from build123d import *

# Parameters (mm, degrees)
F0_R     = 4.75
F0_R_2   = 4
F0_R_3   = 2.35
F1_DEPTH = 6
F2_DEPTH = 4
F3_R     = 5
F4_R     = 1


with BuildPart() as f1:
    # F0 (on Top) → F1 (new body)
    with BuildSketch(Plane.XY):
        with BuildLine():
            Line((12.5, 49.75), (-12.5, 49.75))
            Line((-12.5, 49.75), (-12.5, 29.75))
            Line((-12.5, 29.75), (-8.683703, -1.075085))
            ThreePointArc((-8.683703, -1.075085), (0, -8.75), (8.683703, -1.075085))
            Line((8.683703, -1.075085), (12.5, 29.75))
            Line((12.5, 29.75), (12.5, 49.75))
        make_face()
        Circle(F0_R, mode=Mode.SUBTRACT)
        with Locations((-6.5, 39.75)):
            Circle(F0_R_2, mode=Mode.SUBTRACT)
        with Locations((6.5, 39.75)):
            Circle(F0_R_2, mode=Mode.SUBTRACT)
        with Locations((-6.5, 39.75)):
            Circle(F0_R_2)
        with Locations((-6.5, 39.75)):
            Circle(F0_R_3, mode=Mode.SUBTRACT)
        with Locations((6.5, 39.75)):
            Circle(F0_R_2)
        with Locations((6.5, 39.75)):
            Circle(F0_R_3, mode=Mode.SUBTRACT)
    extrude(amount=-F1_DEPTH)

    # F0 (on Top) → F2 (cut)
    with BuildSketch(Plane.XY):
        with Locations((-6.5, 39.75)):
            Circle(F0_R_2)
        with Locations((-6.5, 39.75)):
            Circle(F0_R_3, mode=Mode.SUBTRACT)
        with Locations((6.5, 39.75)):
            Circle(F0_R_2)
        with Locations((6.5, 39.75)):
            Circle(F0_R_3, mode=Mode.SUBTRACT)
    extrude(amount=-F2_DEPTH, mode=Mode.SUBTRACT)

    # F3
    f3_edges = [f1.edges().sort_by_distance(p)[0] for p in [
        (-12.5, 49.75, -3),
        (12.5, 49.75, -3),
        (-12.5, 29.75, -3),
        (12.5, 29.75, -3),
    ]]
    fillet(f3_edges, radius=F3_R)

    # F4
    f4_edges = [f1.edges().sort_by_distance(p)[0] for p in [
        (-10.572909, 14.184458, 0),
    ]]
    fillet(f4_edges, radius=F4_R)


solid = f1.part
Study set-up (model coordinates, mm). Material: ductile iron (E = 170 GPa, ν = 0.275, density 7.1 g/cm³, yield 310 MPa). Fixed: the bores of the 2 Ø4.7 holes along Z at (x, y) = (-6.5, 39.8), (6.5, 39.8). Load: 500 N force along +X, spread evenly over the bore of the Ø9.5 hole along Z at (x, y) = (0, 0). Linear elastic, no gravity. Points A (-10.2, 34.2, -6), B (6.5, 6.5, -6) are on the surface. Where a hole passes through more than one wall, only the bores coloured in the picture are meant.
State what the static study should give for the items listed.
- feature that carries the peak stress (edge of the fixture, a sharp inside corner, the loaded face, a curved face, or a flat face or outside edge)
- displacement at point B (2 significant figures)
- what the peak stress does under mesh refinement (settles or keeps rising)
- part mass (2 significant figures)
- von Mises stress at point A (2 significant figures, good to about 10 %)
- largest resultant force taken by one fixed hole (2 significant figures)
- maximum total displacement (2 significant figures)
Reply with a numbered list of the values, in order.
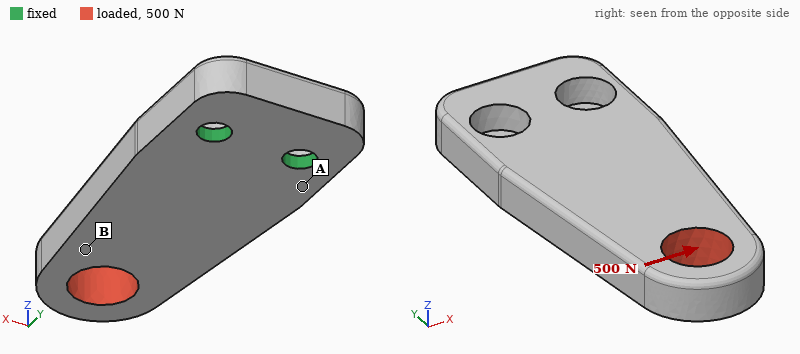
1. edge of the fixture
2. 14 µm
3. keeps rising
4. 46 g
5. 34 MPa
6. 1.3 kN
7. 24 µm
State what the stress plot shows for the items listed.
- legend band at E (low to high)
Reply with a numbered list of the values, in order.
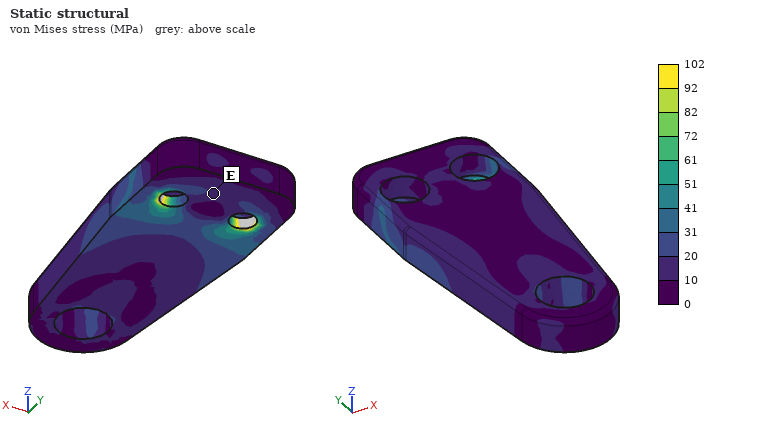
1. 10 to 20 MPa
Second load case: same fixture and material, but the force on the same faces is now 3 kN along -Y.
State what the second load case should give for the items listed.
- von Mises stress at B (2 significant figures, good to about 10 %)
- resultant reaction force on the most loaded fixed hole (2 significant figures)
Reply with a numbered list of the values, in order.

1. 33 MPa
2. 1.5 kN
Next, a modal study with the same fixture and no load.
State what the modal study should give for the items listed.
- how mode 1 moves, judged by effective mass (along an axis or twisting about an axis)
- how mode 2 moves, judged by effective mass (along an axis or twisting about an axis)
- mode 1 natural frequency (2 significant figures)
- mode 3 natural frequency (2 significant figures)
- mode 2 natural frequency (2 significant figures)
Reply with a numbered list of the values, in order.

1. along Z
2. along X
3. 2000 Hz
4. 10 kHz
5. 7300 Hz
